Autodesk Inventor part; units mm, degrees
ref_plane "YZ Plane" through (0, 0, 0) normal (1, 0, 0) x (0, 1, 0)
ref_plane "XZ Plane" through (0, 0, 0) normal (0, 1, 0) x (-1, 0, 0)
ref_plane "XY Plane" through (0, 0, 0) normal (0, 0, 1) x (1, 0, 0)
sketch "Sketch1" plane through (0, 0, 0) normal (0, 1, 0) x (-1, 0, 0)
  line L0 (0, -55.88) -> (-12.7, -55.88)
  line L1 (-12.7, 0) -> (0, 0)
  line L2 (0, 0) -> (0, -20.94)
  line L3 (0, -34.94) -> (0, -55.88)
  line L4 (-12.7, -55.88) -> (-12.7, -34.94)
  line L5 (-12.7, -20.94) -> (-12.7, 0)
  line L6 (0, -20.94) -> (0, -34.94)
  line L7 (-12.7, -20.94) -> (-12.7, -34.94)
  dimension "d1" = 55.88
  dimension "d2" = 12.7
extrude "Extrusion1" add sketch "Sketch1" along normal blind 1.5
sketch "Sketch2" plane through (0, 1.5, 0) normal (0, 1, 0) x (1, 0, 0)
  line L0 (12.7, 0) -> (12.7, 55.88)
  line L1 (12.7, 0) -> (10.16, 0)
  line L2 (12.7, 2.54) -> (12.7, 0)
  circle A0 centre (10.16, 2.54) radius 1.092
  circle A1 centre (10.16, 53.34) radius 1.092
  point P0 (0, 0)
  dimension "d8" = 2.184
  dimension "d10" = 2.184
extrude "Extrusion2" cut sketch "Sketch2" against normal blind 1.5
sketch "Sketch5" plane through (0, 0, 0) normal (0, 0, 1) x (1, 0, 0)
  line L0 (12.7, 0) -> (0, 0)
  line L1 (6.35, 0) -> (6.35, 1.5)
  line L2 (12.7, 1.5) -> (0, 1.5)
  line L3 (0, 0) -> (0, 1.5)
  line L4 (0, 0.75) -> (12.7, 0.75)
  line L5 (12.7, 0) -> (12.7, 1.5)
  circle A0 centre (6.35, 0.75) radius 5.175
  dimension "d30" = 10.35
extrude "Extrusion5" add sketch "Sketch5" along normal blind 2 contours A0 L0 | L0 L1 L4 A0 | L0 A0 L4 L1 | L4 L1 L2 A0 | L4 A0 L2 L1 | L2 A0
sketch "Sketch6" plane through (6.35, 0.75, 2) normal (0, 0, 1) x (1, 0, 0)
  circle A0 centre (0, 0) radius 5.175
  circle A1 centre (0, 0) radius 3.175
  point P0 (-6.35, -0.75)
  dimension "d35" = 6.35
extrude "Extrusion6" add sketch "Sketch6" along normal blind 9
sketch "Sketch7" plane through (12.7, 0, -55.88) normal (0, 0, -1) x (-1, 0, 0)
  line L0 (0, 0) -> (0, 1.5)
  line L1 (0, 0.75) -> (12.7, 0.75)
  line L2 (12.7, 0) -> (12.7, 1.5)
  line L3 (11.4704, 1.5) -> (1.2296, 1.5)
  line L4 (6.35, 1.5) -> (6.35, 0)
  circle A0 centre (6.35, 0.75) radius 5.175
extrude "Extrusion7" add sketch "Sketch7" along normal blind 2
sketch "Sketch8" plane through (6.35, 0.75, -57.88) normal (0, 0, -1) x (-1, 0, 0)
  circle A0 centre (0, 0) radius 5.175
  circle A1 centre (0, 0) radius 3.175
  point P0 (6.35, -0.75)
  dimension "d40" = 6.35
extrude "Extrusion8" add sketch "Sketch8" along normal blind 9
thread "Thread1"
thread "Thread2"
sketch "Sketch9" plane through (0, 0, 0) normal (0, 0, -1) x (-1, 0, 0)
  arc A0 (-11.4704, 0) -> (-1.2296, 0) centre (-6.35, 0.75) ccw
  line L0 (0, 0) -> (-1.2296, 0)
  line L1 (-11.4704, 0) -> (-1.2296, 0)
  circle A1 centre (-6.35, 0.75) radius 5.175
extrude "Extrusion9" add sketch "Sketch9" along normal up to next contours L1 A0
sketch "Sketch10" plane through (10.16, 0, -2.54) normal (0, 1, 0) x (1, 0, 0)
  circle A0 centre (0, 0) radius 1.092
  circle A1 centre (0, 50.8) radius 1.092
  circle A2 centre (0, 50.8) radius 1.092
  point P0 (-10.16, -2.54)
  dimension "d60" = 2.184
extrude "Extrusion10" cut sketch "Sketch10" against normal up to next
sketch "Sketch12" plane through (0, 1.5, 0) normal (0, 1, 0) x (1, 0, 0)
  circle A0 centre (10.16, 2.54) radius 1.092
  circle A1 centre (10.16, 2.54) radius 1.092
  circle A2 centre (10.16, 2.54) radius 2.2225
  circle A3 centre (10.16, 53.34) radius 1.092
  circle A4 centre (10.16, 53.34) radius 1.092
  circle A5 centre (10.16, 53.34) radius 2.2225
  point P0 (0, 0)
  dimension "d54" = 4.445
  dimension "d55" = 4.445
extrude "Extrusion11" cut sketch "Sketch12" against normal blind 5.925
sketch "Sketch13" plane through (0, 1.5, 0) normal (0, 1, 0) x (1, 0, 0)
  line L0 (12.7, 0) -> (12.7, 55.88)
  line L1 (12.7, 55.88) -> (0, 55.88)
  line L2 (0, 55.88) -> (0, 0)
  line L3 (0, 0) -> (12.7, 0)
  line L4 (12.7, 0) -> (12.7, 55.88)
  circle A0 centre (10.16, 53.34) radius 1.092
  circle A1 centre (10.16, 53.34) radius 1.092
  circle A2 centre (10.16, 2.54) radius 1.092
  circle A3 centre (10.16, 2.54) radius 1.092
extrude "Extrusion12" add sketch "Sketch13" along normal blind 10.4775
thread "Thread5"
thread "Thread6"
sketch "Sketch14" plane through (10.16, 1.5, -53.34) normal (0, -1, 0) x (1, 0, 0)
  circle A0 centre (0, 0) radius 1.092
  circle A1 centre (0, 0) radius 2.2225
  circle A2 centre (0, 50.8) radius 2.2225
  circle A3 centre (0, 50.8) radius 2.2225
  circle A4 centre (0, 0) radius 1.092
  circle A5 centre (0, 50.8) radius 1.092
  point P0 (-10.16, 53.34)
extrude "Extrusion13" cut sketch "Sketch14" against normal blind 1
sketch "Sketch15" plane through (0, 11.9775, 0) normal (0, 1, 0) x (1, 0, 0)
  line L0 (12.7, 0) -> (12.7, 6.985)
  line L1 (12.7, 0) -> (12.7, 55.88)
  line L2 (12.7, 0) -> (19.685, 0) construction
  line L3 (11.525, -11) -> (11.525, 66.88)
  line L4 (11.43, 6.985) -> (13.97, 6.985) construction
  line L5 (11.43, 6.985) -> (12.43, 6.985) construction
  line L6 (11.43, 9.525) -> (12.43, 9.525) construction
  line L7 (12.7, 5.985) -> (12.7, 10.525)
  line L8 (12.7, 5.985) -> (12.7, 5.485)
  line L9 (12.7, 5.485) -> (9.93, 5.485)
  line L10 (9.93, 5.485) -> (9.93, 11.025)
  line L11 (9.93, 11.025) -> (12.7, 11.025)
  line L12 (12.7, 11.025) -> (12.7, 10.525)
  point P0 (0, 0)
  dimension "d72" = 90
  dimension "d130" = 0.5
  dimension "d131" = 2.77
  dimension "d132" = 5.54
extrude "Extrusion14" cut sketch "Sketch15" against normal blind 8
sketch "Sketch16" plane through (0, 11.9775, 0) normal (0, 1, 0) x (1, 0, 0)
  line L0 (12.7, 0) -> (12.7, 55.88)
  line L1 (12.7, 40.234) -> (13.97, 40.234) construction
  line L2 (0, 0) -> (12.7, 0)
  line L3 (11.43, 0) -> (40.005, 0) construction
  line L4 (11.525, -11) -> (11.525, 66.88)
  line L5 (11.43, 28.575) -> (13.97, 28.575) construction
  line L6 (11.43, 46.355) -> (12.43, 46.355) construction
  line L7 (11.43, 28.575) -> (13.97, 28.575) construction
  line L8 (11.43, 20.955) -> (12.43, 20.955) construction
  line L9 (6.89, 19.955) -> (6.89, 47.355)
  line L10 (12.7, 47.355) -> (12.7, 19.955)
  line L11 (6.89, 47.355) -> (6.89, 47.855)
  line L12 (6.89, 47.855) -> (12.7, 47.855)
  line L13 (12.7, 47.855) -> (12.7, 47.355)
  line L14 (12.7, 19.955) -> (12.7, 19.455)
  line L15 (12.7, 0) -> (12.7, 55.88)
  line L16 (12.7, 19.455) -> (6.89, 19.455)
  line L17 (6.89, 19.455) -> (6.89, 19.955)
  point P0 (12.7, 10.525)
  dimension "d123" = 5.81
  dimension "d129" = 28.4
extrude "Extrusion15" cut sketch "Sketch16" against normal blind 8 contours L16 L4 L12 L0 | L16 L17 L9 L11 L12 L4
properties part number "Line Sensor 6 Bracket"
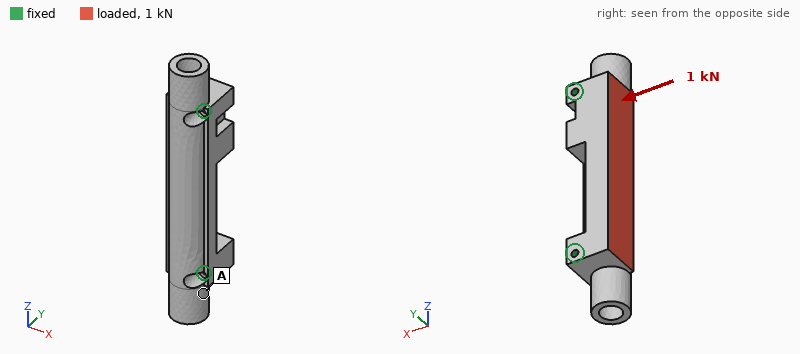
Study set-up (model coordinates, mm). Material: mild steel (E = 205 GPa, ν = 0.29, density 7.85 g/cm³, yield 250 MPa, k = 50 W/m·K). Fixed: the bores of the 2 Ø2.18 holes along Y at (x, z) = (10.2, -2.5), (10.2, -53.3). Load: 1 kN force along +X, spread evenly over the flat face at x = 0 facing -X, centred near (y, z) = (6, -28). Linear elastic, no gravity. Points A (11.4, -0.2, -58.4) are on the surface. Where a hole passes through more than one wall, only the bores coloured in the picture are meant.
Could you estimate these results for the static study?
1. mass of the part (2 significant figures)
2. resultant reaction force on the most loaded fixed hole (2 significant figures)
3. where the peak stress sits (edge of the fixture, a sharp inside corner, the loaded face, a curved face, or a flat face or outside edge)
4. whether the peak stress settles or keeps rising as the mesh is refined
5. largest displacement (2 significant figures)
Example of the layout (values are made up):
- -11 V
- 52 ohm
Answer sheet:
- 79 g
- 650 N
- edge of the fixture
- keeps rising
- 3.3 µm
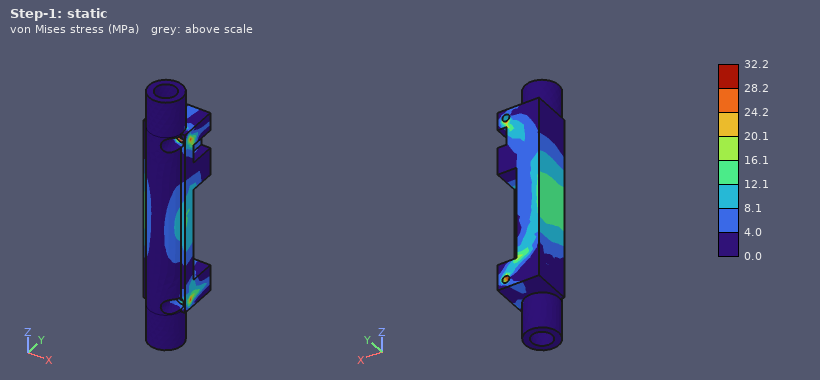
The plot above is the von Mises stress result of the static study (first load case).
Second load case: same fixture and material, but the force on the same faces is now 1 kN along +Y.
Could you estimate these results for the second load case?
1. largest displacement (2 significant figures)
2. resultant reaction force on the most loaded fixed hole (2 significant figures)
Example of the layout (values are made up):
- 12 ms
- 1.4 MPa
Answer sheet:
- 4.9 µm
- 530 N
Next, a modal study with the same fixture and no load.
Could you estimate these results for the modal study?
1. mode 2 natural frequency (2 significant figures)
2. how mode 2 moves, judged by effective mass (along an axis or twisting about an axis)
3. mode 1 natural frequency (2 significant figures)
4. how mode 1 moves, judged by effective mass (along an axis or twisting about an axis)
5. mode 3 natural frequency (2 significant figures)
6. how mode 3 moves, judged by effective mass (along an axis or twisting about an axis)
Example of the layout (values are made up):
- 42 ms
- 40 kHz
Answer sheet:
- 14 kHz
- along Y
- 12 kHz
- along X
- 18 kHz
- twisting about Z
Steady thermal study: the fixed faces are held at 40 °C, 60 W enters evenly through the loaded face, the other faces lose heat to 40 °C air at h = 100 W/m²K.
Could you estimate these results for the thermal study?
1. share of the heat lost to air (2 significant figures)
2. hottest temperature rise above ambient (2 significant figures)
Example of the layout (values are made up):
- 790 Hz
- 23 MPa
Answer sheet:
- 20 %
- 65 K
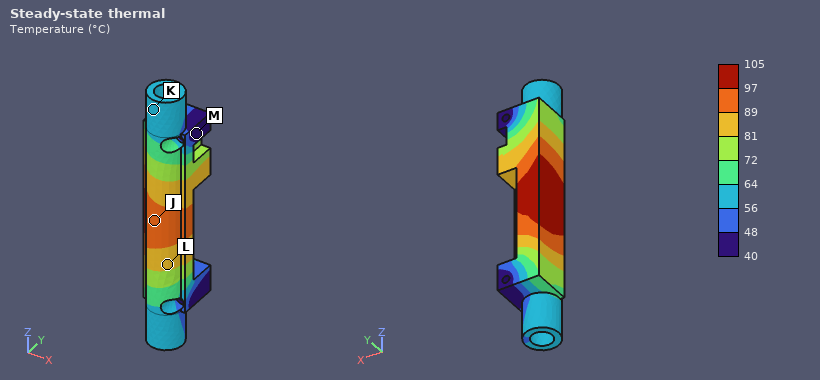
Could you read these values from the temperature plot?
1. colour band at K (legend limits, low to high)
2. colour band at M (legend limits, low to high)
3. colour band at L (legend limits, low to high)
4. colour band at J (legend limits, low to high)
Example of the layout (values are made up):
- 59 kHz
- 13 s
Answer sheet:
- 56 to 64 °C
- 40 to 48 °C
- 81 to 89 °C
- 89 to 97 °C
